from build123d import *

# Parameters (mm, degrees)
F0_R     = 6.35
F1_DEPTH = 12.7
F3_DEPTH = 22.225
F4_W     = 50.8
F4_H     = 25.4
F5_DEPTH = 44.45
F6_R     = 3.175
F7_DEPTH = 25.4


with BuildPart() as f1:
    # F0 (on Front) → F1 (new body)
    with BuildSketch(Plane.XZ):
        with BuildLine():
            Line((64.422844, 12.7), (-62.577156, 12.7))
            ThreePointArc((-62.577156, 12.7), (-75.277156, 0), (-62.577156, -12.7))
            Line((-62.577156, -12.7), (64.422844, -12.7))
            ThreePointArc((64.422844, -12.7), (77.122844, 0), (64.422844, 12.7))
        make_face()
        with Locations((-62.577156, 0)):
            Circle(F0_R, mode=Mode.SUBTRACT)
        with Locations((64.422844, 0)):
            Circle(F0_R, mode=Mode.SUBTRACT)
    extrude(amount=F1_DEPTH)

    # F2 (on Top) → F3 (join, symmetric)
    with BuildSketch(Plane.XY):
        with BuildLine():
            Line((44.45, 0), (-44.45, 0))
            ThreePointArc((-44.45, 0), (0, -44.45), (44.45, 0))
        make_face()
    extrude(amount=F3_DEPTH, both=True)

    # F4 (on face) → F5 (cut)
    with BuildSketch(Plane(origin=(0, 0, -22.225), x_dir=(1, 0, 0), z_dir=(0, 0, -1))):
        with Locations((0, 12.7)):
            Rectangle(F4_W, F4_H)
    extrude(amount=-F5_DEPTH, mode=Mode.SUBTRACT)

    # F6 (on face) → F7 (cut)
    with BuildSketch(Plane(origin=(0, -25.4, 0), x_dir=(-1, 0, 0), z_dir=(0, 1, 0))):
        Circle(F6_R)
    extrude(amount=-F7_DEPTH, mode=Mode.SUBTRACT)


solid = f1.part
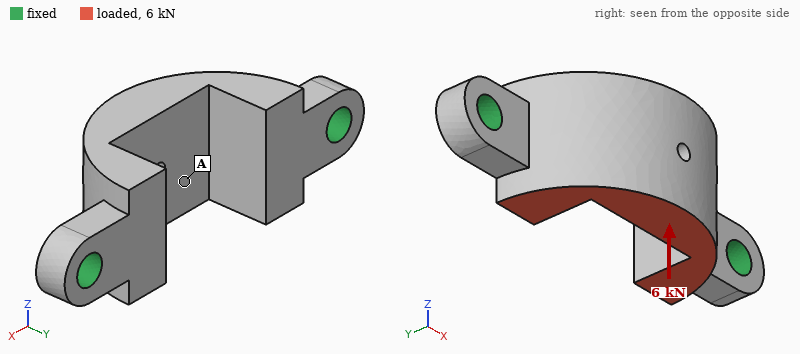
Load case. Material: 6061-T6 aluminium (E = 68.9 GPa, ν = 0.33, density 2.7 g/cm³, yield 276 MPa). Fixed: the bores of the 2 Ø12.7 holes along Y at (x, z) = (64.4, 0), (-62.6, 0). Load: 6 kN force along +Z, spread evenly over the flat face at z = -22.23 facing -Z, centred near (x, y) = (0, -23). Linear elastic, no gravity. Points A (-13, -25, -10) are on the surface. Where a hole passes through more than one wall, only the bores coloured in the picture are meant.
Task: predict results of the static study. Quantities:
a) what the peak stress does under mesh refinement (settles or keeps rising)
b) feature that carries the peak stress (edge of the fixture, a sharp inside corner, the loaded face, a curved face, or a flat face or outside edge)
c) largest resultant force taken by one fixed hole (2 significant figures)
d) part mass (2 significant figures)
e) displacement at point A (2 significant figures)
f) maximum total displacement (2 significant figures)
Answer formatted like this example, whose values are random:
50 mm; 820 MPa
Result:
keeps rising; edge of the fixture; 3.1 kN; 260 g; 0.095 mm; 0.17 mm
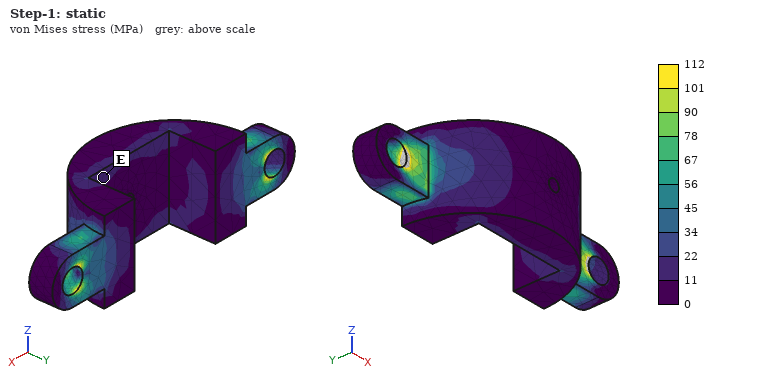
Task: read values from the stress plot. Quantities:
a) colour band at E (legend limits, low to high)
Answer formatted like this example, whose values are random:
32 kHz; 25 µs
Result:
11 to 22 MPa
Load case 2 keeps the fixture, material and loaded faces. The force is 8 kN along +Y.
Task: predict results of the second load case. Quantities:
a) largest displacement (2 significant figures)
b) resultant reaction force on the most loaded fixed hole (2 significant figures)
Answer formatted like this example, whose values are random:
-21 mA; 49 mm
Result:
0.26 mm; 5.2 kN
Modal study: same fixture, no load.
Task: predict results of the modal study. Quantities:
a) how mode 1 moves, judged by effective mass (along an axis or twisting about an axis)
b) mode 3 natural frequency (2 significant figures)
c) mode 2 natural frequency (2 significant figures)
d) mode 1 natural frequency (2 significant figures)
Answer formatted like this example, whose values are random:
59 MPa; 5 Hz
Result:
along Z; 5700 Hz; 5500 Hz; 2400 Hz
